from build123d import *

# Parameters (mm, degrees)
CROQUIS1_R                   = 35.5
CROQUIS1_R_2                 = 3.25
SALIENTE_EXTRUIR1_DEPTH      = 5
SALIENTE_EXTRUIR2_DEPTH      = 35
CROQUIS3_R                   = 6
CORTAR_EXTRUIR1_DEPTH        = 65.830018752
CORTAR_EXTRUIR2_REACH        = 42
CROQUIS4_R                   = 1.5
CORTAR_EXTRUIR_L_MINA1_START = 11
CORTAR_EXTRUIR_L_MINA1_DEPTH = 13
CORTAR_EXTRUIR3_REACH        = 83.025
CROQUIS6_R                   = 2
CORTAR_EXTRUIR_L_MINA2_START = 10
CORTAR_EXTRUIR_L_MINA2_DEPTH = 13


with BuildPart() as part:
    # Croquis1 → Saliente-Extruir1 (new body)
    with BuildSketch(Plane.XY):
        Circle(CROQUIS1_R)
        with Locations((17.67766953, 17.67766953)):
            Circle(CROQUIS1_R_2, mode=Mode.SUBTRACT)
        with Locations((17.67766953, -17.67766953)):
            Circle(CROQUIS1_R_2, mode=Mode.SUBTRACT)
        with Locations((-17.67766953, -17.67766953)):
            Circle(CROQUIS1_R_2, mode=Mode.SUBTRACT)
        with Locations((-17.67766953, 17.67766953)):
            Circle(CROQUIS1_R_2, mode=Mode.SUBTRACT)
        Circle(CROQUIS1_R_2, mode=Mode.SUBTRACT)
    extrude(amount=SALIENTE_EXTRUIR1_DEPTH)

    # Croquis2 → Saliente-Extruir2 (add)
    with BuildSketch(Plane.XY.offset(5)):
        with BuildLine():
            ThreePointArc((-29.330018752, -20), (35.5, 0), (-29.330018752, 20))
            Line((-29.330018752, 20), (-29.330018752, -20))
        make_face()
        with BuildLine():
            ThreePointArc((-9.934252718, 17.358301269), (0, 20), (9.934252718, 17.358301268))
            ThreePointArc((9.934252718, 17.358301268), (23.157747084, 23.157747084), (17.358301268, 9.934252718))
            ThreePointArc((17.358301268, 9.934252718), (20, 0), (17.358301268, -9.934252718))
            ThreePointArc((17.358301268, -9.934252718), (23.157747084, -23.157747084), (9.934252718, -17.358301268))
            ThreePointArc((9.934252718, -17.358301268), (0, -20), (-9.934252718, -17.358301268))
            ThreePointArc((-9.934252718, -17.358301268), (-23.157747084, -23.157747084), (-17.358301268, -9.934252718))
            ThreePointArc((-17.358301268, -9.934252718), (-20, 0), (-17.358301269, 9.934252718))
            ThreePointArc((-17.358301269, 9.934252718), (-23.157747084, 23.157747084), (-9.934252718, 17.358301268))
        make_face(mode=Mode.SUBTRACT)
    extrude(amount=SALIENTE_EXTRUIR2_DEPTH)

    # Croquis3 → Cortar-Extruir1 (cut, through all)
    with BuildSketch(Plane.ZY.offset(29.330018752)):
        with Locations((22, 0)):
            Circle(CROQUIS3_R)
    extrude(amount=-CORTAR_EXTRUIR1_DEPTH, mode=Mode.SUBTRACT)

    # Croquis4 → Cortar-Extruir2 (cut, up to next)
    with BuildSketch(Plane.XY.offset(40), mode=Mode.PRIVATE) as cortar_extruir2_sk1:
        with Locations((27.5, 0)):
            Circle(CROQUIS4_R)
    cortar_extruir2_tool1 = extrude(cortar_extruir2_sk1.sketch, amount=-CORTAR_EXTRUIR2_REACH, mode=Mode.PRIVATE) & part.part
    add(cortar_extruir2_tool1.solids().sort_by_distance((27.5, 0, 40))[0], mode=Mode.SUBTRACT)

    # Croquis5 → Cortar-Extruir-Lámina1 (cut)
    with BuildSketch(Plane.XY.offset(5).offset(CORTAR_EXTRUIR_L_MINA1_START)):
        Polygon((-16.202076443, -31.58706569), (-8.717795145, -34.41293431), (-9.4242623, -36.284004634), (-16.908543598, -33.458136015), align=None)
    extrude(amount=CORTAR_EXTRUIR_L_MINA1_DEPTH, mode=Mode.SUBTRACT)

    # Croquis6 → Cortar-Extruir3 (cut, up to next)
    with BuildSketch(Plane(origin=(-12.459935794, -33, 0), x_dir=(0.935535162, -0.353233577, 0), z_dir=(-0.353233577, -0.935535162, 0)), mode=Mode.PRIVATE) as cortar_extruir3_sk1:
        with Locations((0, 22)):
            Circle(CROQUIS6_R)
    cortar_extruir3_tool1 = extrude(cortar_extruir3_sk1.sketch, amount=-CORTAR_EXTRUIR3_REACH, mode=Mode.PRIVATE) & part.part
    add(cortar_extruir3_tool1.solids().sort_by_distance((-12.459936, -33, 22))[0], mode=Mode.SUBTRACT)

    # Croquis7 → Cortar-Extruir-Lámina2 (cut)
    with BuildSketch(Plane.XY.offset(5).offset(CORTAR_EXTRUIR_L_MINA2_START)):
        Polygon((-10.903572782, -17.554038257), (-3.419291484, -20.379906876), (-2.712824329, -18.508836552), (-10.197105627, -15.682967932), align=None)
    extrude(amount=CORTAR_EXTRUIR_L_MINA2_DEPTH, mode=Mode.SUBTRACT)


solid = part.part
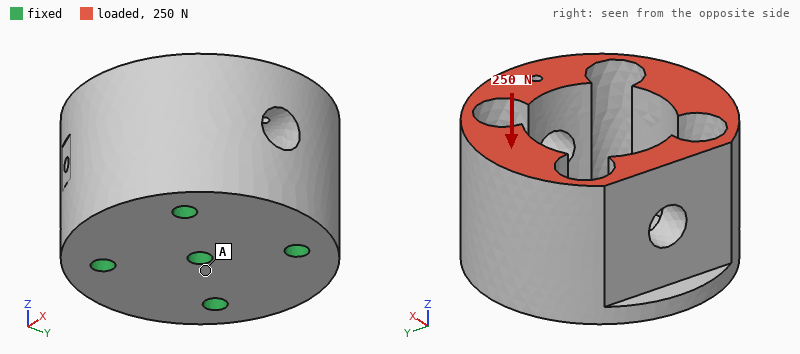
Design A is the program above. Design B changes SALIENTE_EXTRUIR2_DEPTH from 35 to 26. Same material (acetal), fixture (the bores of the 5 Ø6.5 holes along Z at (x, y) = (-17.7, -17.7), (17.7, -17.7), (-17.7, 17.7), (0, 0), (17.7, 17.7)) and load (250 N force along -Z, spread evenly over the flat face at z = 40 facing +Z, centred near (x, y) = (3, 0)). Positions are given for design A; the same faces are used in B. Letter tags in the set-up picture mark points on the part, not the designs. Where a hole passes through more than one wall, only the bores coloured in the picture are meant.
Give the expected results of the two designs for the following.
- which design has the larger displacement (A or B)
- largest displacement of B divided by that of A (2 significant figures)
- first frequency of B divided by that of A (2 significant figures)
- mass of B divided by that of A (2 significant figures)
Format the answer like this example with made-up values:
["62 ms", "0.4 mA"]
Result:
["B", "1.3", "1.2", "0.79"]
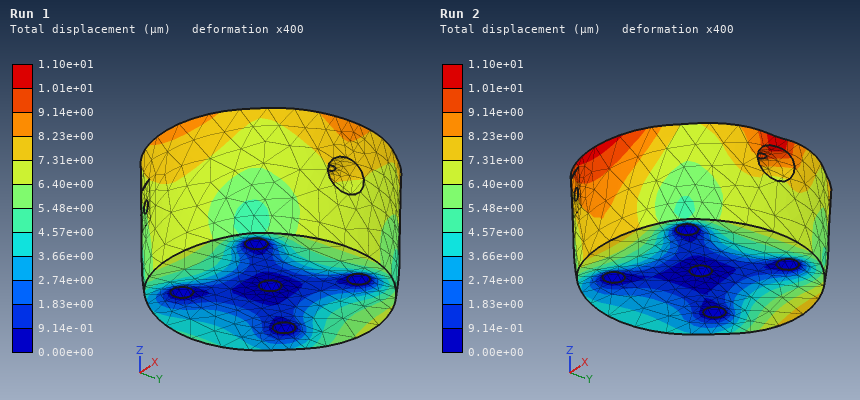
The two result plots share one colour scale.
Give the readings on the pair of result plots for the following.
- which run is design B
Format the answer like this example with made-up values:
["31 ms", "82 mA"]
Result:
["Run 2"]
